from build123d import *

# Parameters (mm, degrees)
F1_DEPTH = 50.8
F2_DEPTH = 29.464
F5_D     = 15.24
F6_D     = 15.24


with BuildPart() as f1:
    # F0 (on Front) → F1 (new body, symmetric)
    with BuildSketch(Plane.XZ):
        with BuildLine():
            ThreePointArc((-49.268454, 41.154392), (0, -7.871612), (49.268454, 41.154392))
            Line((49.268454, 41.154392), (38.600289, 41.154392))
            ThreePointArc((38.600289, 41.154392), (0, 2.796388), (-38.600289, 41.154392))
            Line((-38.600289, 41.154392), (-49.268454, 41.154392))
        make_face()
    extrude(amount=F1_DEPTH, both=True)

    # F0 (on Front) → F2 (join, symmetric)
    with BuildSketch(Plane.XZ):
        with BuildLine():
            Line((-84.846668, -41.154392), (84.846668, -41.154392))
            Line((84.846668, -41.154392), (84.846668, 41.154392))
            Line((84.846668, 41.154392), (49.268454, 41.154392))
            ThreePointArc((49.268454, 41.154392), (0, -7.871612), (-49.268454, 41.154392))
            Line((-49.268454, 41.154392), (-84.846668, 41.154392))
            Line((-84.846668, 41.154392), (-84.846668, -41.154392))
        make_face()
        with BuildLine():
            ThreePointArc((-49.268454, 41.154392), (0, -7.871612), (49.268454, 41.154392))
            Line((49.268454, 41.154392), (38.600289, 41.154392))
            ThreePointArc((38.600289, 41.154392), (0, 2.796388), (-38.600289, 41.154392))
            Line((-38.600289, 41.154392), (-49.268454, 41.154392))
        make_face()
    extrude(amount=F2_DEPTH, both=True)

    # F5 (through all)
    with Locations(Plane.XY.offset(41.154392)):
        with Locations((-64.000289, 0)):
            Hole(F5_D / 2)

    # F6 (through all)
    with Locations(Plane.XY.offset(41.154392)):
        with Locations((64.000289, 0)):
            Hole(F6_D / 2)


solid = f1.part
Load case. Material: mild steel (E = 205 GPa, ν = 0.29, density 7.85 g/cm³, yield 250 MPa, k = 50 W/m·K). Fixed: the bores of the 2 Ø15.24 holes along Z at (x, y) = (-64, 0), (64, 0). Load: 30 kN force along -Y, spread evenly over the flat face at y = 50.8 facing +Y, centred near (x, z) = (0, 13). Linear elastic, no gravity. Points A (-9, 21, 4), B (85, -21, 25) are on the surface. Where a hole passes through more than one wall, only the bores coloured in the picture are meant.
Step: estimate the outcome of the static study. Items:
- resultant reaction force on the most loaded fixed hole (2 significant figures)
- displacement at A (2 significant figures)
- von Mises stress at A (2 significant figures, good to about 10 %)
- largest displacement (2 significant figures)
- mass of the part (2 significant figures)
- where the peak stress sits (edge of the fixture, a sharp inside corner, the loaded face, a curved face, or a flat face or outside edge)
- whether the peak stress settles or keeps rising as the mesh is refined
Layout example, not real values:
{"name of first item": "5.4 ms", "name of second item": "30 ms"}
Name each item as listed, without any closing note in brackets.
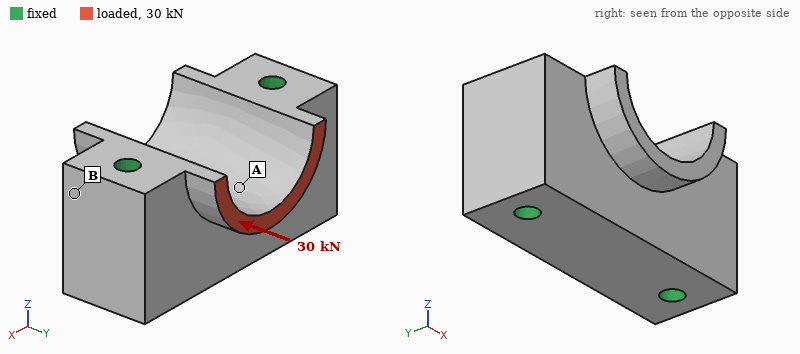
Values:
{"resultant reaction force on the most loaded fixed hole": "15 kN", "displacement at A": "4.1 µm", "von Mises stress at A": "11 MPa", "largest displacement": "8.4 µm", "mass of the part": "5.6 kg", "where the peak stress sits": "edge of the fixture", "whether the peak stress settles or keeps rising as the mesh is refined": "keeps rising"}
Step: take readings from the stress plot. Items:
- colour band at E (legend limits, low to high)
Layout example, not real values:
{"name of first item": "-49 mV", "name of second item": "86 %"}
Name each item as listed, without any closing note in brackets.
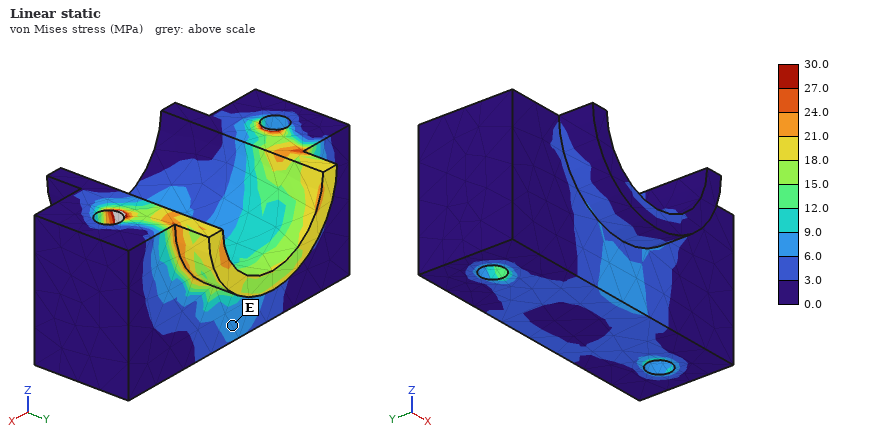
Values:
{"colour band at E": "6.0 to 9.0 MPa"}
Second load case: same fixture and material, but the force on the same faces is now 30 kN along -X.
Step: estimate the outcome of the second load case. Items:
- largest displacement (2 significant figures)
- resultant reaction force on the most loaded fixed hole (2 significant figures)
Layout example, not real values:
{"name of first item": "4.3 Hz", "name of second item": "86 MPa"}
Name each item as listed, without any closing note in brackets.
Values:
{"largest displacement": "57 µm", "resultant reaction force on the most loaded fixed hole": "19 kN"}
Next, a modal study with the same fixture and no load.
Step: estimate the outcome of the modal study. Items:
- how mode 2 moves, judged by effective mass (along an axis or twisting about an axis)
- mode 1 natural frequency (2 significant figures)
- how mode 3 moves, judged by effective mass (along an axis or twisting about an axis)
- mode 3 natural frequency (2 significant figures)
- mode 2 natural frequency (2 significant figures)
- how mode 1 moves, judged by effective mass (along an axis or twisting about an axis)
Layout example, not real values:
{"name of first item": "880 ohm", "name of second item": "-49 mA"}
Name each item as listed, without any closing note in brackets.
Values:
{"how mode 2 moves, judged by effective mass": "along Z", "mode 1 natural frequency": "8300 Hz", "how mode 3 moves, judged by effective mass": "twisting about X", "mode 3 natural frequency": "11 kHz", "mode 2 natural frequency": "10 kHz", "how mode 1 moves, judged by effective mass": "along Y"}
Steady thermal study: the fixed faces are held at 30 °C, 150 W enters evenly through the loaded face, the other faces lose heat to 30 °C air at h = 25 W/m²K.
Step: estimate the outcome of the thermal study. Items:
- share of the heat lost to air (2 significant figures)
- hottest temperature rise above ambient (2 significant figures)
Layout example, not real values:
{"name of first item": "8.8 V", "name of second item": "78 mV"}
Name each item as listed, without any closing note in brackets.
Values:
{"share of the heat lost to air": "9.9 %", "hottest temperature rise above ambient": "72 K"}
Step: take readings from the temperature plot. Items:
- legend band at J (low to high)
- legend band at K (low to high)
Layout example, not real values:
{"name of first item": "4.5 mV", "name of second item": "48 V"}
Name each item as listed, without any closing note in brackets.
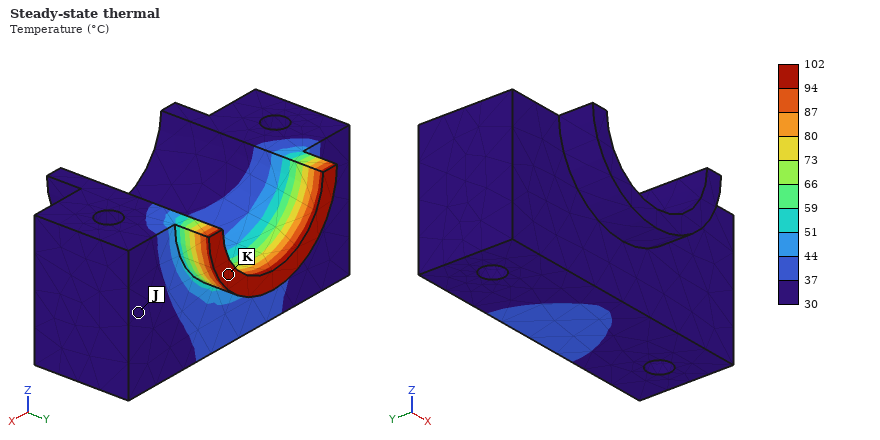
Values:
{"legend band at J": "30 to 37 °C", "legend band at K": "94 to 102 °C"}
